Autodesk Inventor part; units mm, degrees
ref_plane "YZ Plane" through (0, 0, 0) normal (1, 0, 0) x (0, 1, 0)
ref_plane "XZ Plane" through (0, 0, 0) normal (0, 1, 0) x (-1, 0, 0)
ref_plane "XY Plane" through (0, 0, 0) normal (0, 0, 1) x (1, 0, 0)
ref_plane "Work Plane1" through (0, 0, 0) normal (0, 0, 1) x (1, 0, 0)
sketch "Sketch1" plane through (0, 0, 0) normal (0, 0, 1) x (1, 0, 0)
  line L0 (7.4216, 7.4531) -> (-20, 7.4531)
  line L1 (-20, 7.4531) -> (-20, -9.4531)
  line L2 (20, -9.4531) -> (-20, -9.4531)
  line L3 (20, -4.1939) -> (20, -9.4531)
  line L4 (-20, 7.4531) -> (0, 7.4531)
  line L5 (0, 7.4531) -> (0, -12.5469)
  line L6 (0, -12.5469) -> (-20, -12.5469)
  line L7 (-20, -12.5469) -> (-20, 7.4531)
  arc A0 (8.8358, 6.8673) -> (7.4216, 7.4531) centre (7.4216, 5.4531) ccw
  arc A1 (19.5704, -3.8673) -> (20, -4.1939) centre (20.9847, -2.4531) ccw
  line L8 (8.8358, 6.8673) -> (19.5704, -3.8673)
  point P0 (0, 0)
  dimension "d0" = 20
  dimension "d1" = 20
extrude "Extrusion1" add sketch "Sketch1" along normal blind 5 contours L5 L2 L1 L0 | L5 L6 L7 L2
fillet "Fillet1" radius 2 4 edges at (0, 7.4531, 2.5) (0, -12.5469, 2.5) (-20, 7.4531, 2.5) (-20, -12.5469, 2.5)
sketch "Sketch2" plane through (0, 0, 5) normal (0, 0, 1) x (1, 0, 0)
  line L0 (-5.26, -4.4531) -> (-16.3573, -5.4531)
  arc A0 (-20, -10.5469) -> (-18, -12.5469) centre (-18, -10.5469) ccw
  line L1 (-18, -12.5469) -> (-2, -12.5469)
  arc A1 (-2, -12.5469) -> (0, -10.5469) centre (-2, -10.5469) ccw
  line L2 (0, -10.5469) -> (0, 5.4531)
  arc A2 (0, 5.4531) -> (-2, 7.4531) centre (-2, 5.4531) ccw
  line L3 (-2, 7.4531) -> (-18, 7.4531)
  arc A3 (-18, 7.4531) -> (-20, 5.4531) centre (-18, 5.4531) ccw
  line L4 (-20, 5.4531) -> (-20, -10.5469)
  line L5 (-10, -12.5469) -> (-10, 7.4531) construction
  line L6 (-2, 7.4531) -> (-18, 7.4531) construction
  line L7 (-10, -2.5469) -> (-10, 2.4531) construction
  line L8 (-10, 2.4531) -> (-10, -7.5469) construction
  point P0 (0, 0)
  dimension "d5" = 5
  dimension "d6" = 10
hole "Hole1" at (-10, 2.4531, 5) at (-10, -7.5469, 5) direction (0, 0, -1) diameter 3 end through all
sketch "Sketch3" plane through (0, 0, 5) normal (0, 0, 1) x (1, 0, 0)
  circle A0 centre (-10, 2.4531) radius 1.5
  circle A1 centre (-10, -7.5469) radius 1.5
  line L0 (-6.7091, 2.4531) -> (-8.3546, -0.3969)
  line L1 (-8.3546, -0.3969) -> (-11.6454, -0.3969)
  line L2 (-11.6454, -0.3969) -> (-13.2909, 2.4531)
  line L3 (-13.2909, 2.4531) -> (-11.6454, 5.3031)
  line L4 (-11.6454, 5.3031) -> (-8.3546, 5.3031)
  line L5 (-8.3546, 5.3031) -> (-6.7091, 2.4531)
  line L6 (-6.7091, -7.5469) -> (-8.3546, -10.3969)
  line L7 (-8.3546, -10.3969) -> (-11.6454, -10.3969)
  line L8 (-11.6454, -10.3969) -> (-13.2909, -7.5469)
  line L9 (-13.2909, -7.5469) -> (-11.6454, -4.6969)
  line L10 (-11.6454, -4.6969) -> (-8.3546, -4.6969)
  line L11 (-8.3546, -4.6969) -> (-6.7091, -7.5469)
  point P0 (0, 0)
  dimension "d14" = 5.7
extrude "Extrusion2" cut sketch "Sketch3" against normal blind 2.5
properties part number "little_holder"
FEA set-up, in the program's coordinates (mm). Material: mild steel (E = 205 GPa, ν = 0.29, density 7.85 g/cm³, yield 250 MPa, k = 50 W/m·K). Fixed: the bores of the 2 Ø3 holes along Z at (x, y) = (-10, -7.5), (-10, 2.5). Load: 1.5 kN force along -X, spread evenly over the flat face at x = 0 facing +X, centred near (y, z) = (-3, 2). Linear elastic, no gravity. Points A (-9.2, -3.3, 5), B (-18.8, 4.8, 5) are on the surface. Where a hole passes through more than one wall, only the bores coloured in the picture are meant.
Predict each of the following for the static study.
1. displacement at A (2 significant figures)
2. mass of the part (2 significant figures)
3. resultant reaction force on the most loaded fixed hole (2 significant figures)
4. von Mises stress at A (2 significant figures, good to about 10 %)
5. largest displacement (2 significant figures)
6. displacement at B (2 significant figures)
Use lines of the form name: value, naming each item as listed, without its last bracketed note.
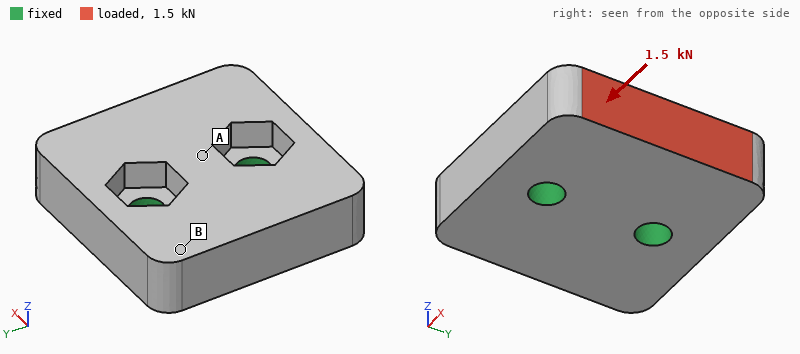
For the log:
displacement at A: 1.7 µm
mass of the part: 14 g
resultant reaction force on the most loaded fixed hole: 760 N
von Mises stress at A: 23 MPa
largest displacement: 4.6 µm
displacement at B: 2.7 µm
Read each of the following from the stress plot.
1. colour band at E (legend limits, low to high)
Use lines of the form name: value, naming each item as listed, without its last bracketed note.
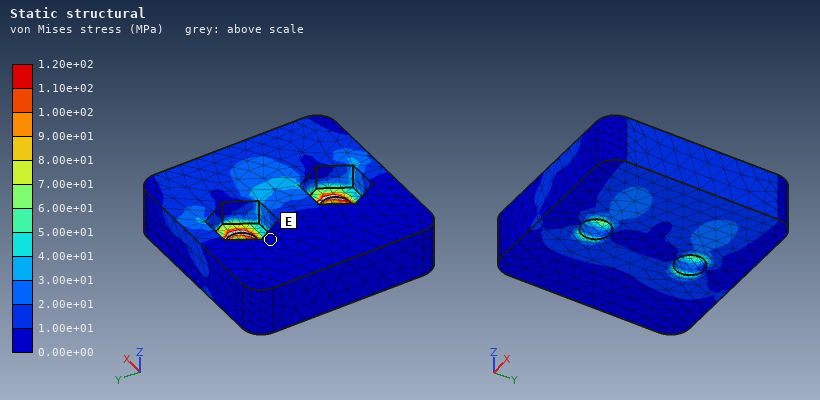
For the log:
colour band at E: 0.00e+00 to 1.00e+01 MPa
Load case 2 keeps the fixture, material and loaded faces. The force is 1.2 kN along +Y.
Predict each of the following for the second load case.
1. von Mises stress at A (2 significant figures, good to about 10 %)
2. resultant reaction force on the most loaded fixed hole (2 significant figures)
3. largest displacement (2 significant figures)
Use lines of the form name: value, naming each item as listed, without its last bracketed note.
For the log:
von Mises stress at A: 13 MPa
resultant reaction force on the most loaded fixed hole: 1.1 kN
largest displacement: 4.1 µm
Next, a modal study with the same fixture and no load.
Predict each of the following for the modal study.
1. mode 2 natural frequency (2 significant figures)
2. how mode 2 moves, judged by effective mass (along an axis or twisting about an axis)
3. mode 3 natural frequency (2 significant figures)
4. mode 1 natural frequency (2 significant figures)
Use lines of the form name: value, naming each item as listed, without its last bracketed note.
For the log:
mode 2 natural frequency: 31 kHz
how mode 2 moves, judged by effective mass: along Z
mode 3 natural frequency: 35 kHz
mode 1 natural frequency: 18 kHz
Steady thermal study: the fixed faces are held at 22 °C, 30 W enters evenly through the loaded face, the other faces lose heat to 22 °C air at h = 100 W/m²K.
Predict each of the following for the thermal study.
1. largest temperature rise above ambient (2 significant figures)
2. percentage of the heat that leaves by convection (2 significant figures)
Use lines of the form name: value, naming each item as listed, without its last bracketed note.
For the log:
largest temperature rise above ambient: 76 K
percentage of the heat that leaves by convection: 8.6 %
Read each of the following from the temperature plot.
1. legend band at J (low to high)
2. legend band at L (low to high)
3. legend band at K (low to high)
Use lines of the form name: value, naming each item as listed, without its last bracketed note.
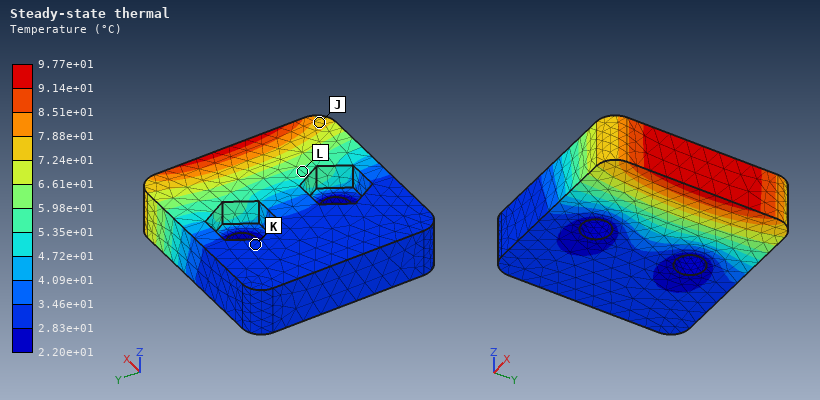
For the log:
legend band at J: 7.24e+01 to 7.88e+01 °C
legend band at L: 5.35e+01 to 5.98e+01 °C
legend band at K: 2.83e+01 to 3.46e+01 °C
